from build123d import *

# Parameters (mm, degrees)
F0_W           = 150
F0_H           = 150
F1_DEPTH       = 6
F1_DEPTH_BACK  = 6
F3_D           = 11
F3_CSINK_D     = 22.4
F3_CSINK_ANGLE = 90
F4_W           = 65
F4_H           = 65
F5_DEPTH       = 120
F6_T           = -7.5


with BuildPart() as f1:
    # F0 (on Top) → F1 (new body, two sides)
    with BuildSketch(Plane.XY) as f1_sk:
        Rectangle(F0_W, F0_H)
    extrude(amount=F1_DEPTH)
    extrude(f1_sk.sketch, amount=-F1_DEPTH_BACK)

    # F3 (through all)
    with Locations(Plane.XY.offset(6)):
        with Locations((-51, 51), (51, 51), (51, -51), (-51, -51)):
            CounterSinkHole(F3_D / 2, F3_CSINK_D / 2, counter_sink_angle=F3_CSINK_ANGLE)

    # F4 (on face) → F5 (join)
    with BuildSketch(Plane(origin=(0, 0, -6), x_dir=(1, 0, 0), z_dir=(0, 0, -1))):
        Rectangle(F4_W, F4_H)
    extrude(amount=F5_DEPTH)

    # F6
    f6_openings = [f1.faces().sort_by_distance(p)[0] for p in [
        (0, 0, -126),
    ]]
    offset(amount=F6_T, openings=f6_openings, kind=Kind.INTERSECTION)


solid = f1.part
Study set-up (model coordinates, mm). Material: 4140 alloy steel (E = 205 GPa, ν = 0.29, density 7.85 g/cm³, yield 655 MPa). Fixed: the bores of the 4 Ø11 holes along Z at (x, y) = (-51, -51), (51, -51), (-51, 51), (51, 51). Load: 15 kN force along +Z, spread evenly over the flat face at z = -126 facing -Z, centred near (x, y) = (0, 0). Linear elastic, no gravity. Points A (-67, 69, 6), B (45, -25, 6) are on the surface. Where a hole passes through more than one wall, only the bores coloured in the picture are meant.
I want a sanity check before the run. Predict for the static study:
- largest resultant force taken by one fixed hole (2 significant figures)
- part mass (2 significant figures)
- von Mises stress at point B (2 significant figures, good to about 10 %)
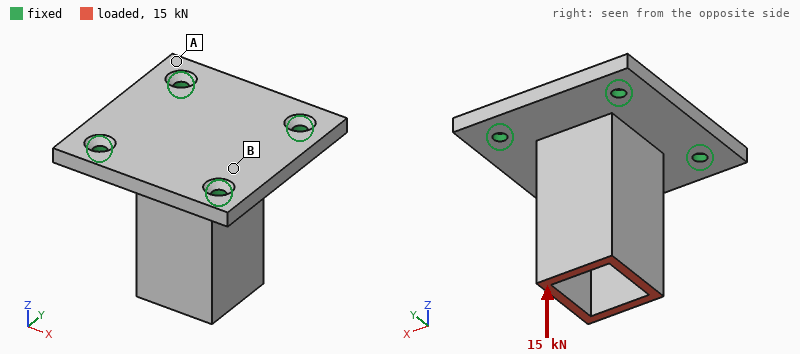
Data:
4.4 kN
3.6 kg
24 MPa
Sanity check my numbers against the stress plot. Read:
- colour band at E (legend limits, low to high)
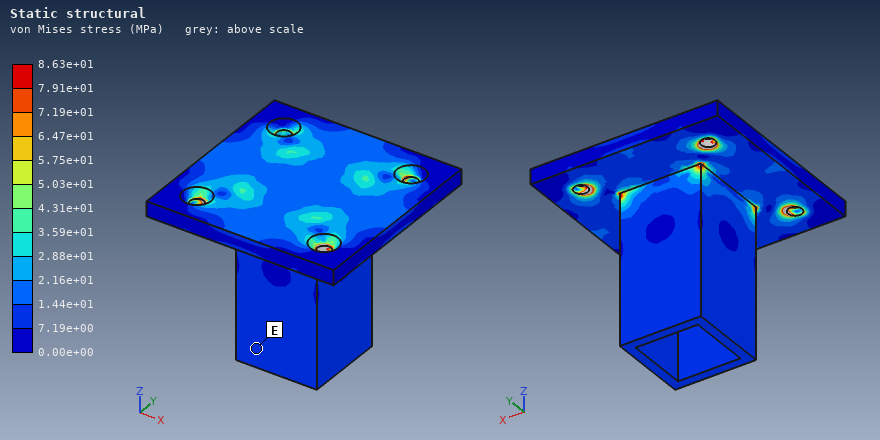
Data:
7.19e+00 to 1.44e+01 MPa
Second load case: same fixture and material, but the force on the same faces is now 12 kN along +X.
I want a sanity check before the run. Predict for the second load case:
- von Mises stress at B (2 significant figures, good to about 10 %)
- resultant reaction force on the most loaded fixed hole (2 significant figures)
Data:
52 MPa
8.8 kN
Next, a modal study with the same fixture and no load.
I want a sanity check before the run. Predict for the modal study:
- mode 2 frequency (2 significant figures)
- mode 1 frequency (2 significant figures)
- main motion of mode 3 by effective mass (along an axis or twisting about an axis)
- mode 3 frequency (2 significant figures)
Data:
1600 Hz
1600 Hz
along Z
2600 Hz
